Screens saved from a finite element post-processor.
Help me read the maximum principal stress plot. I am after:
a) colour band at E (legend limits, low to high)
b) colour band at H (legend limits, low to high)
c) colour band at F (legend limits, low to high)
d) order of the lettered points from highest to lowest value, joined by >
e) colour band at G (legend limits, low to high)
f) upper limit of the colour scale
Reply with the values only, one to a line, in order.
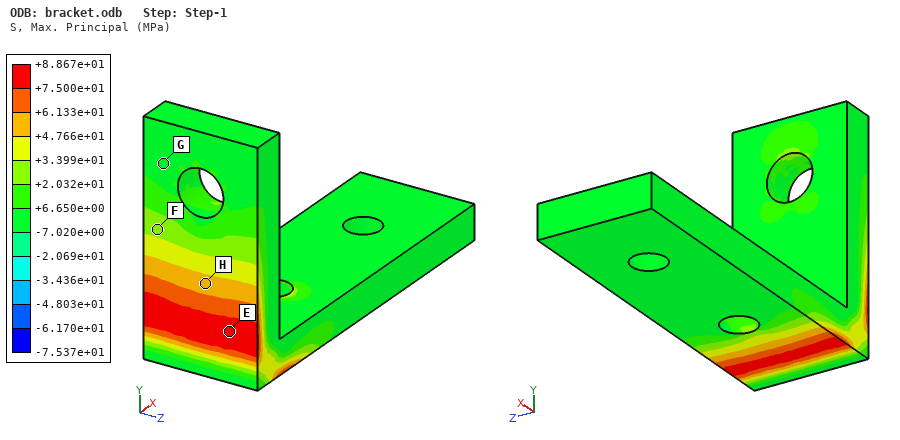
+7.500e+01 to +8.867e+01 MPa
+4.766e+01 to +6.133e+01 MPa
+2.032e+01 to +3.399e+01 MPa
E > H > F > G
-7.020e+00 to +6.650e+00 MPa
+8.867e+01 MPa
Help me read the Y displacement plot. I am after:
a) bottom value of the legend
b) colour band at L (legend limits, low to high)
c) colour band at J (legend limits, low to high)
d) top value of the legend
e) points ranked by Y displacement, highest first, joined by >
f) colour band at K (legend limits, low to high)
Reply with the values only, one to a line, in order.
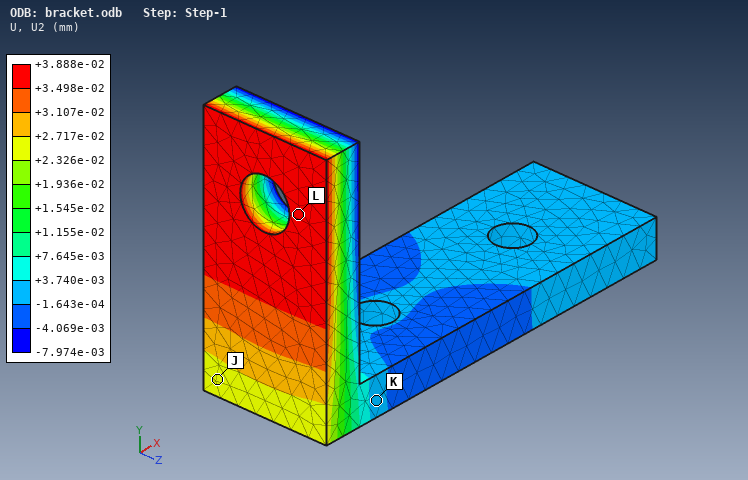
-7.974e-03 mm
+3.498e-02 to +3.888e-02 mm
+2.326e-02 to +2.717e-02 mm
+3.888e-02 mm
L > J > K
-1.643e-04 to +3.740e-03 mm
